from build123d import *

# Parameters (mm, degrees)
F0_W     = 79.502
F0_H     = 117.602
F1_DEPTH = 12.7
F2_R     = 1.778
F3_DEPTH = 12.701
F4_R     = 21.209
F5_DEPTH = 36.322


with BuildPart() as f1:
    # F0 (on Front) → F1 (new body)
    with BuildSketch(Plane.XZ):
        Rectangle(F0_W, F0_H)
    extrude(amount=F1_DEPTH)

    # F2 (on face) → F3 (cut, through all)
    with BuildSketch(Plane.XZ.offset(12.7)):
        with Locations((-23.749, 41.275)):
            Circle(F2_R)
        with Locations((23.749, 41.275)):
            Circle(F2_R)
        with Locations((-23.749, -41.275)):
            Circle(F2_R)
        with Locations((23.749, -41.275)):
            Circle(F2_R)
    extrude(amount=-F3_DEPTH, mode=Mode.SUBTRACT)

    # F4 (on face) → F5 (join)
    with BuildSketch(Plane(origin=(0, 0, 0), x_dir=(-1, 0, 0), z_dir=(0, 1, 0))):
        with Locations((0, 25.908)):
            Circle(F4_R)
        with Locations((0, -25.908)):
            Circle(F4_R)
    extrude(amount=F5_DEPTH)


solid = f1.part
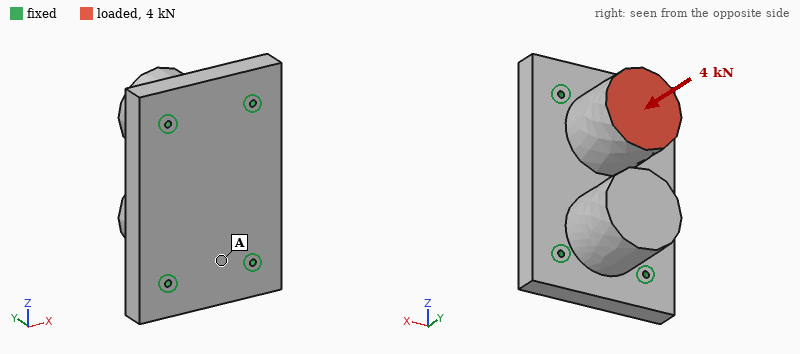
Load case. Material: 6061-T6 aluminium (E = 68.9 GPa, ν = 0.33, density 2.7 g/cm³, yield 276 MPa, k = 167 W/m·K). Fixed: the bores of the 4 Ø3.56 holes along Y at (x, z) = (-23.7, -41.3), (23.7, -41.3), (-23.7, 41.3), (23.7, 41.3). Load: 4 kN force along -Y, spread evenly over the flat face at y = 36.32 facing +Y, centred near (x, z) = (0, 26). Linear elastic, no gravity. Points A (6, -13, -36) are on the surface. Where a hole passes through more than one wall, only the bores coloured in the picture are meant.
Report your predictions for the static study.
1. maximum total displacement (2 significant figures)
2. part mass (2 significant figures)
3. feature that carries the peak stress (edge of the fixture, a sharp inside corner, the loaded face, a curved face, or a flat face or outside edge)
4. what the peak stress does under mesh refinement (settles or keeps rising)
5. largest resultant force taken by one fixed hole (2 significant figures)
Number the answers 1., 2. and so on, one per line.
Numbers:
1. 16 µm
2. 600 g
3. edge of the fixture
4. keeps rising
5. 1.7 kN
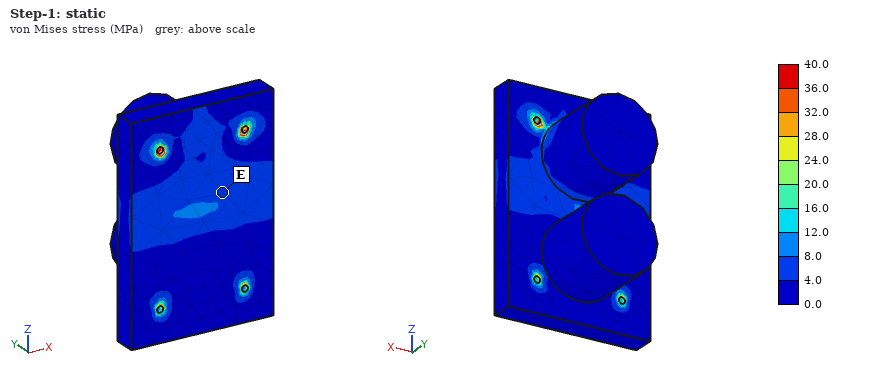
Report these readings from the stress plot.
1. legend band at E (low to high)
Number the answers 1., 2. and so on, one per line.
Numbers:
1. 4.0 to 8.0 MPa
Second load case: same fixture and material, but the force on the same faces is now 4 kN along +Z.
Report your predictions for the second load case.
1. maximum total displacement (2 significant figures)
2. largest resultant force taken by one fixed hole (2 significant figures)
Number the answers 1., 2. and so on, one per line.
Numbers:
1. 59 µm
2. 1.7 kN
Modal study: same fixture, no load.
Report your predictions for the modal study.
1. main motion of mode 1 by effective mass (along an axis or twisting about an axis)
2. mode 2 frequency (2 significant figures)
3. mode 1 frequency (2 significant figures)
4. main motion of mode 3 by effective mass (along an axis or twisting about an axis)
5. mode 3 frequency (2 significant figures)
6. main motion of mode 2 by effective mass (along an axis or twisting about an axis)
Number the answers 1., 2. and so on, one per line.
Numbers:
1. along Y
2. 6600 Hz
3. 3800 Hz
4. along Z
5. 7900 Hz
6. along X
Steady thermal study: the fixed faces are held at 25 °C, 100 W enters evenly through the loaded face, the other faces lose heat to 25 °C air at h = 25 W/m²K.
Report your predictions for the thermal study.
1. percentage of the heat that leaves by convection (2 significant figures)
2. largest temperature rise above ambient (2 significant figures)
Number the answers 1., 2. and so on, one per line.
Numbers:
1. 4.8 %
2. 26 K
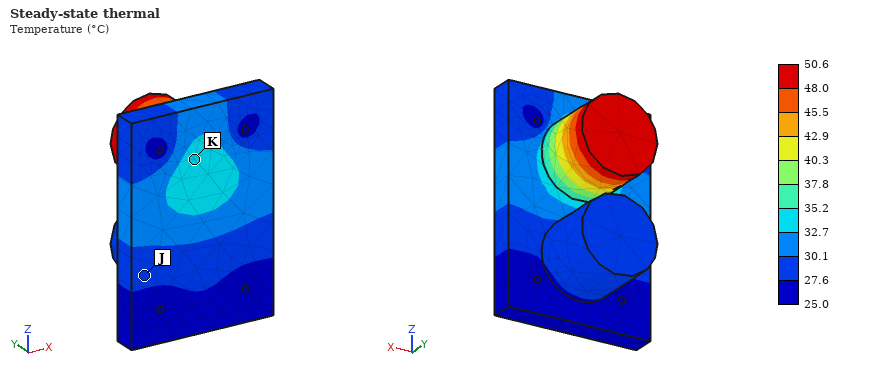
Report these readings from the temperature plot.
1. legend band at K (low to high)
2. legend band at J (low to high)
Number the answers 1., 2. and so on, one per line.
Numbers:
1. 32.7 to 35.2 °C
2. 27.6 to 30.1 °C
